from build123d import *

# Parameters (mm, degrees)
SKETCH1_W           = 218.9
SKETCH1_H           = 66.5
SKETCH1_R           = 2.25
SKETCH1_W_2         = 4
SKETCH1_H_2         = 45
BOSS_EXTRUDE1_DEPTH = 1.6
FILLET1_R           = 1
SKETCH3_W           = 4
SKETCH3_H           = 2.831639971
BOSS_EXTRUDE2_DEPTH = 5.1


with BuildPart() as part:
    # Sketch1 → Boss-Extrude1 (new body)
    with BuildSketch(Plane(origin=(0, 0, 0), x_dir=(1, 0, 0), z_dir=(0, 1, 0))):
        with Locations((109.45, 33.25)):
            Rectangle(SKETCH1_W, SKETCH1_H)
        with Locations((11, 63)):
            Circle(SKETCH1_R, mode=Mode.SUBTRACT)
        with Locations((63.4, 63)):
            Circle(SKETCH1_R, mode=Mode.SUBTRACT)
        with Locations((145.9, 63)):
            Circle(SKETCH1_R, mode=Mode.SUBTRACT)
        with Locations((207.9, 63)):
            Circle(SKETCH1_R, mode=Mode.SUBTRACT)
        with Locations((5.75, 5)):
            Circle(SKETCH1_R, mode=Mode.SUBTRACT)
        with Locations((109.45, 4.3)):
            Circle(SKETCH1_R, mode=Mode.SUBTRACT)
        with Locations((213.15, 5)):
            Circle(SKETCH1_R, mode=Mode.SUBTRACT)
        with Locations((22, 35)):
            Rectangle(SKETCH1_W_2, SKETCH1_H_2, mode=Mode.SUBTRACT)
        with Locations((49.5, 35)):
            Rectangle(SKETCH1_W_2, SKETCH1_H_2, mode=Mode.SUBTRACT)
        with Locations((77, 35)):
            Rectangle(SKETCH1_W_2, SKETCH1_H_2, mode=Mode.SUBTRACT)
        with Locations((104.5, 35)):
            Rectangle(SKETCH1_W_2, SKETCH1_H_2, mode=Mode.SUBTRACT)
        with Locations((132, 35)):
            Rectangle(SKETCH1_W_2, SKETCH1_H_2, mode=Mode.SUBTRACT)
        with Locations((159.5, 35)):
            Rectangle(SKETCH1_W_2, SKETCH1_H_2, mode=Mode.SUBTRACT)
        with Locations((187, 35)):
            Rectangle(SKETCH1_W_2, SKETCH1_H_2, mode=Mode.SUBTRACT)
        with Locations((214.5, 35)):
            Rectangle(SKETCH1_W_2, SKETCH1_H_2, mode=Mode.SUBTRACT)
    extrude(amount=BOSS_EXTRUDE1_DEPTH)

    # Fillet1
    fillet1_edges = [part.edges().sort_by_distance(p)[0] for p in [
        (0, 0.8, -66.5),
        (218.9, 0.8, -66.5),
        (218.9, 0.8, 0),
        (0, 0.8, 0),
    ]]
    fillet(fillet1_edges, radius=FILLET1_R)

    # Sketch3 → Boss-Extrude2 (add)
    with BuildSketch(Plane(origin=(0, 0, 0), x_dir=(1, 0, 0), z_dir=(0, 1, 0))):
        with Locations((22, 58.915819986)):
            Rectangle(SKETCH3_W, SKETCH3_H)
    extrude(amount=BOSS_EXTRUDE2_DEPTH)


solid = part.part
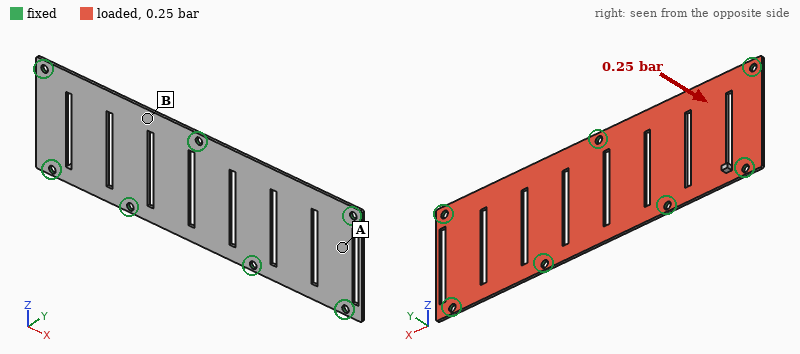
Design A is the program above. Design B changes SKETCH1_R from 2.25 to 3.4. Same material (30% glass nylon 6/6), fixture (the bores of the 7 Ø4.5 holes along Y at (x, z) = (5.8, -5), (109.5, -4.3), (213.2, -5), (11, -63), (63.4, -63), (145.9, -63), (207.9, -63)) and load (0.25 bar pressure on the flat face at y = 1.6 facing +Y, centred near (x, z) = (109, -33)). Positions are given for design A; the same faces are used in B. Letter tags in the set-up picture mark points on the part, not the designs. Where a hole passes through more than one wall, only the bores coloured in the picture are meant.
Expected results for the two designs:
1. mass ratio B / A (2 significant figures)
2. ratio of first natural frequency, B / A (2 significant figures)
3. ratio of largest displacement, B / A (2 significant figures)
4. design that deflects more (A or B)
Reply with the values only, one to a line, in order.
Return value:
0.99
1.1
0.89
A
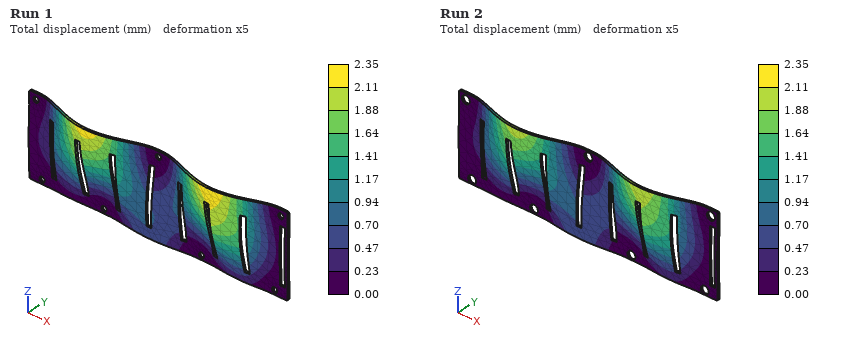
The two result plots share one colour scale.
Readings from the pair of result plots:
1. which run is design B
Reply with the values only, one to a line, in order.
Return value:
Run 2
